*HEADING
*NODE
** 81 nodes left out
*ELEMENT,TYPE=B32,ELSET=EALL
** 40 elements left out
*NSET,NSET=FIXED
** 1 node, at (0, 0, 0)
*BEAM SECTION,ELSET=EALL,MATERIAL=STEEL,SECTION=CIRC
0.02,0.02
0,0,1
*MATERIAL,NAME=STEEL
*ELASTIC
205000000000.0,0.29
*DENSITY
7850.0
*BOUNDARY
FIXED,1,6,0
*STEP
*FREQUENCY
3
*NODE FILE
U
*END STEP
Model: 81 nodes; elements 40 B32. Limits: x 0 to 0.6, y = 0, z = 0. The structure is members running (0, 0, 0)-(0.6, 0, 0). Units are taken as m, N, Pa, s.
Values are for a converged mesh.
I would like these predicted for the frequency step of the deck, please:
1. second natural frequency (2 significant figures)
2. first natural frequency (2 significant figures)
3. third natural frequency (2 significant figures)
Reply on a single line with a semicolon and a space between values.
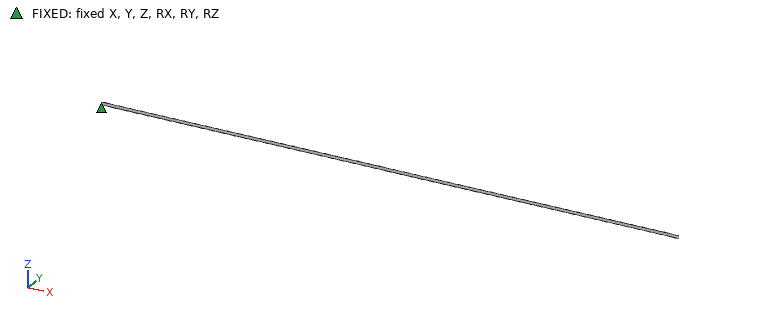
40 Hz; 40 Hz; 250 Hz
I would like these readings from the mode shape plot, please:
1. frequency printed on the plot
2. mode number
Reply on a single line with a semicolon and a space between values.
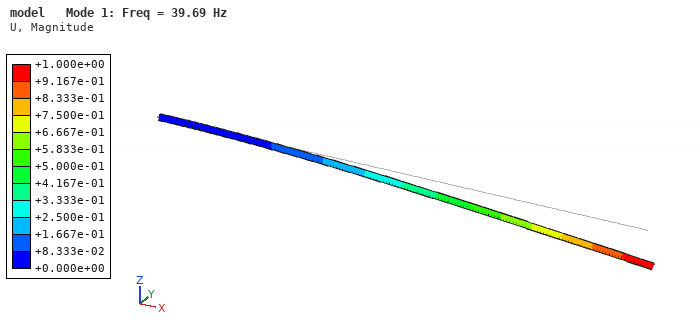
39.69 Hz; 1
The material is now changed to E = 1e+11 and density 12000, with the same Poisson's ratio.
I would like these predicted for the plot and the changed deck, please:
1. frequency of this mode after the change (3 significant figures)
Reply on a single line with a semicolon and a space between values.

22.4 Hz
